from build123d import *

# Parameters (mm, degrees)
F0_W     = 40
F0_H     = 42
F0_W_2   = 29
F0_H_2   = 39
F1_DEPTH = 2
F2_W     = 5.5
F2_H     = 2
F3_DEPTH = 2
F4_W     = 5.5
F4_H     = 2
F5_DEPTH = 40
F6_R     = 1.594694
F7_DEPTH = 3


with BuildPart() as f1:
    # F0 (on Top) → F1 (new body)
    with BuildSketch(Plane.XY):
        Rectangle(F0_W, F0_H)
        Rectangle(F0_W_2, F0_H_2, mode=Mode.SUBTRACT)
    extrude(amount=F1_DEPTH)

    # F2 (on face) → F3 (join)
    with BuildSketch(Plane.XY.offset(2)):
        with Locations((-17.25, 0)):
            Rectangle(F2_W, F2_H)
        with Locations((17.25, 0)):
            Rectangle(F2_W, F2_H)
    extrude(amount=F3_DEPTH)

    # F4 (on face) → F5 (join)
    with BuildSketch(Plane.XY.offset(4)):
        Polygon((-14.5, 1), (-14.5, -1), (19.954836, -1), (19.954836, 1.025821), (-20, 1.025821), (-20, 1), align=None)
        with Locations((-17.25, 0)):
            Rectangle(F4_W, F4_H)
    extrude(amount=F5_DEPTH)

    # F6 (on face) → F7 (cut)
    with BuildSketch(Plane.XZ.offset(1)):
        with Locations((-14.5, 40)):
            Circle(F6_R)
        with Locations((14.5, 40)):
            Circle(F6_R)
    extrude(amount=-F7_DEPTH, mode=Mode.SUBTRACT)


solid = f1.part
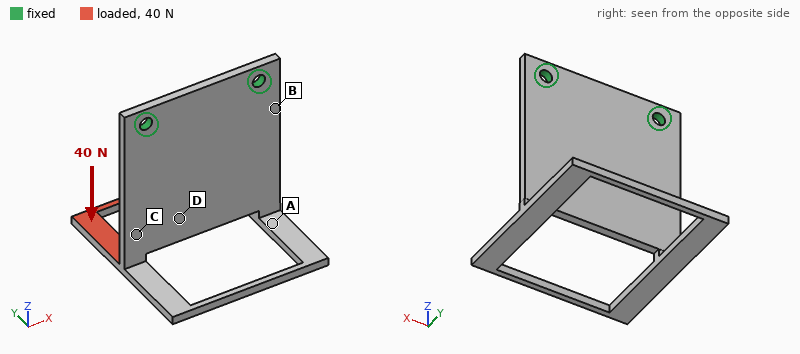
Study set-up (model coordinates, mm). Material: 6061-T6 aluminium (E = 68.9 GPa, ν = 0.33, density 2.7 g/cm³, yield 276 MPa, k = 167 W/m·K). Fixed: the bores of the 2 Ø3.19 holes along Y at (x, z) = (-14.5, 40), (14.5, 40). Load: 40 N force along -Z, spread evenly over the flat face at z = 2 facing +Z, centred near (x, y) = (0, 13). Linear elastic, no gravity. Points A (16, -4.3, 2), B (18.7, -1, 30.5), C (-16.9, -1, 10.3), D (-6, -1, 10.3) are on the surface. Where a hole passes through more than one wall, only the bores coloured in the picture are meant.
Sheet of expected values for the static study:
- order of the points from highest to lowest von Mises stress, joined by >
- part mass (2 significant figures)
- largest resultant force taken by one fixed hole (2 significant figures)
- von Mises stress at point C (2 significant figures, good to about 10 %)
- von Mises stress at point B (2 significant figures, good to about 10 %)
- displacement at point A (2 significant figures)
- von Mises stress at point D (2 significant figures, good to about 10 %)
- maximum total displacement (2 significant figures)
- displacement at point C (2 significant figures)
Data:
C > B > D > A
12 g
20 N
28 MPa
21 MPa
0.22 mm
13 MPa
0.51 mm
0.12 mm
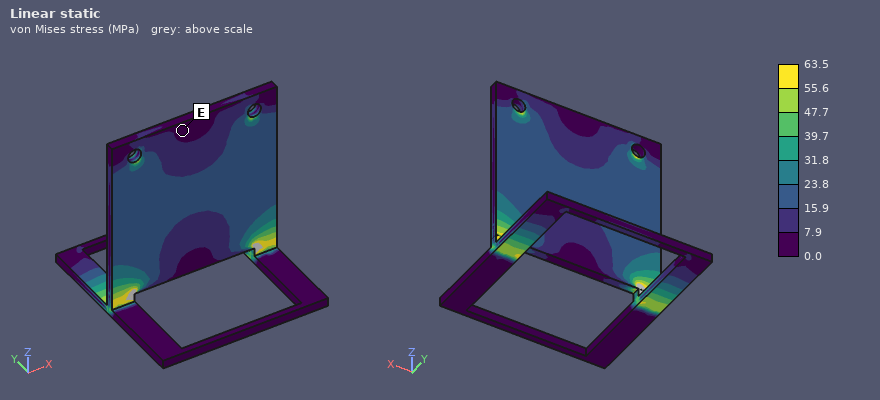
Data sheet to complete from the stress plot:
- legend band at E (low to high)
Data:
0.0 to 7.9 MPa
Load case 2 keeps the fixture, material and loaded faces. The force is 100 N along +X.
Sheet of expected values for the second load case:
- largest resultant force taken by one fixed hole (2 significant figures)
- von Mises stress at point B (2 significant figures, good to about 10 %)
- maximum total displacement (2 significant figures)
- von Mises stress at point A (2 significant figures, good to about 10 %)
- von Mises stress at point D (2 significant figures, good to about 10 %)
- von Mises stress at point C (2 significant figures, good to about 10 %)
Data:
140 N
35 MPa
0.53 mm
14 MPa
23 MPa
67 MPa
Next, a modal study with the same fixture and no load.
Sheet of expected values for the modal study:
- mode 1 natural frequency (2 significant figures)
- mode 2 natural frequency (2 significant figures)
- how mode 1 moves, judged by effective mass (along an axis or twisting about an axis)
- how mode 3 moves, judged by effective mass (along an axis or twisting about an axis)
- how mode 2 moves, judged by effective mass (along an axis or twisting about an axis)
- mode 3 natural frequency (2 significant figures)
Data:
640 Hz
1200 Hz
along Y
along Y
twisting about Z
1700 Hz
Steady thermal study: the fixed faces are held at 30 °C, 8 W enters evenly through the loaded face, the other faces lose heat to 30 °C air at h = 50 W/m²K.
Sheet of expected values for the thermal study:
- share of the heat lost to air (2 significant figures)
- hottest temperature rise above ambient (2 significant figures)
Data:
42 %
53 K
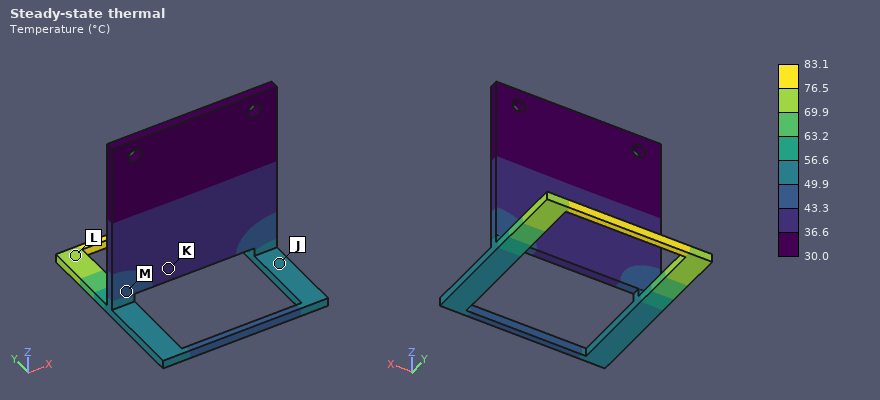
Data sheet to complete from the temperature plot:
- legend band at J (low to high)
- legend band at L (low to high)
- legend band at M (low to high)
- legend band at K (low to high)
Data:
49.9 to 56.6 °C
69.9 to 76.5 °C
43.3 to 49.9 °C
36.6 to 43.3 °C
